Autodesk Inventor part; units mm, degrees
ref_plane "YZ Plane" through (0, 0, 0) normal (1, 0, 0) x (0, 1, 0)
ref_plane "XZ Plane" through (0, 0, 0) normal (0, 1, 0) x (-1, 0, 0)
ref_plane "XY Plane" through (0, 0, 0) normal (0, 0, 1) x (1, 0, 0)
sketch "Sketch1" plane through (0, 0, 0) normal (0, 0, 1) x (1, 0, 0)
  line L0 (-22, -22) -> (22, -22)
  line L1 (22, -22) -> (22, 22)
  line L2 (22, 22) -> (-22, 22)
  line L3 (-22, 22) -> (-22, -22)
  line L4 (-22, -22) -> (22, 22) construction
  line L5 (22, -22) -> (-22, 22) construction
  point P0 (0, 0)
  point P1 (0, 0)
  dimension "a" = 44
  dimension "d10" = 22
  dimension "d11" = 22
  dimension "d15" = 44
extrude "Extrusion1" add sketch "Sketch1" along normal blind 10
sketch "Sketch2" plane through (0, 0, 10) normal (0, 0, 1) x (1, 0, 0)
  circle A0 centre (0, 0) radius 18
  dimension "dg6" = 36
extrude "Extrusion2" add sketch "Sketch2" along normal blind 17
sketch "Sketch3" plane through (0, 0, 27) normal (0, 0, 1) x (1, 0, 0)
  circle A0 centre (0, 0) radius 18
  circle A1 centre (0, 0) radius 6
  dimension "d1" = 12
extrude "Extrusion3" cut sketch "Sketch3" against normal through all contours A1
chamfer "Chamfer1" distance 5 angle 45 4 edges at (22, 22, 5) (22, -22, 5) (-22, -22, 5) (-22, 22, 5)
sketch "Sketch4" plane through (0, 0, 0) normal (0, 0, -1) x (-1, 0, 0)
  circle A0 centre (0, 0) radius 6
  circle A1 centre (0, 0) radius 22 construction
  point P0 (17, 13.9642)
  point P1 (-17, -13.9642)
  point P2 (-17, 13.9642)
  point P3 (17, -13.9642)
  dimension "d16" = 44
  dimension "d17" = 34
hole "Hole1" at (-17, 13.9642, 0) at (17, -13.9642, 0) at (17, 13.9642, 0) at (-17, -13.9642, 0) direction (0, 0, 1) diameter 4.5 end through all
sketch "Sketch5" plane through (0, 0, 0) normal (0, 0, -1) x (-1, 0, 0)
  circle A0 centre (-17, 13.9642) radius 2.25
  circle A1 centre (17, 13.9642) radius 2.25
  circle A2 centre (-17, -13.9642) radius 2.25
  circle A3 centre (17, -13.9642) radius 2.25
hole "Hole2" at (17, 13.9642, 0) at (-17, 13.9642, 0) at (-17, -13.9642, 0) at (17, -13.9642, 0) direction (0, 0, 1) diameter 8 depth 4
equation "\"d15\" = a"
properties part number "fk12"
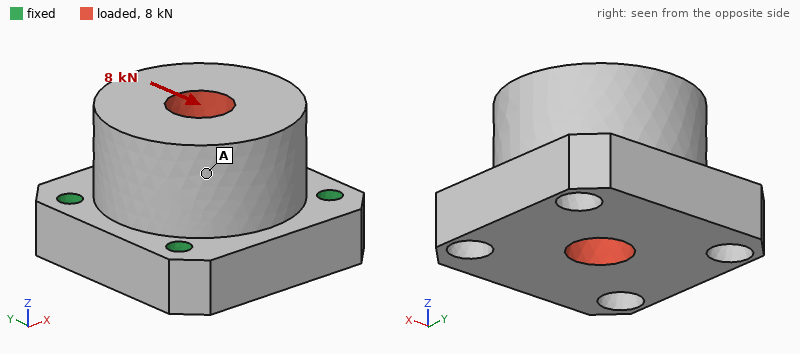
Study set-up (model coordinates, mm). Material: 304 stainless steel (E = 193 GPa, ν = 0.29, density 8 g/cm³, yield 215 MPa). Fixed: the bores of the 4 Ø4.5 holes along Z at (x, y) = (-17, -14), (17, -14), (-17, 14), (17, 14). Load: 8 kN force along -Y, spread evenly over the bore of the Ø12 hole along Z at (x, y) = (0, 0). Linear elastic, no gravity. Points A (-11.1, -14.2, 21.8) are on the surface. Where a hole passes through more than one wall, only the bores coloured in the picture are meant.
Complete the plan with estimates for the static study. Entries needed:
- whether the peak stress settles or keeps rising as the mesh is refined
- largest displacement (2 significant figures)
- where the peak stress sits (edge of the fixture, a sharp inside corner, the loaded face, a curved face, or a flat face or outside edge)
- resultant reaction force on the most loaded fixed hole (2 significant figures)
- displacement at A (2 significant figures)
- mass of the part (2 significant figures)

keeps rising
4.6 µm
edge of the fixture
2.3 kN
3.6 µm
260 g
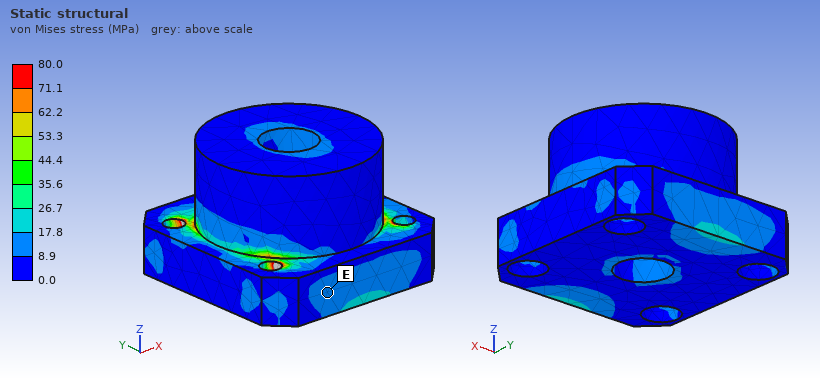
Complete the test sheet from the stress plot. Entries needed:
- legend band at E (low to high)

8.9 to 17.8 MPa
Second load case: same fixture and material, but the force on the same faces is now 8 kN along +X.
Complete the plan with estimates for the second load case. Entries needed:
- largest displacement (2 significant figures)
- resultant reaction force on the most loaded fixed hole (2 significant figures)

3.7 µm
2.2 kN
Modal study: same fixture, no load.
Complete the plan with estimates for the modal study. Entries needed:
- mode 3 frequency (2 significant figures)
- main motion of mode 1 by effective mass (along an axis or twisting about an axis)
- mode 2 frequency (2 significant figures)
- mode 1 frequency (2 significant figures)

19 kHz
along Y
19 kHz
17 kHz
